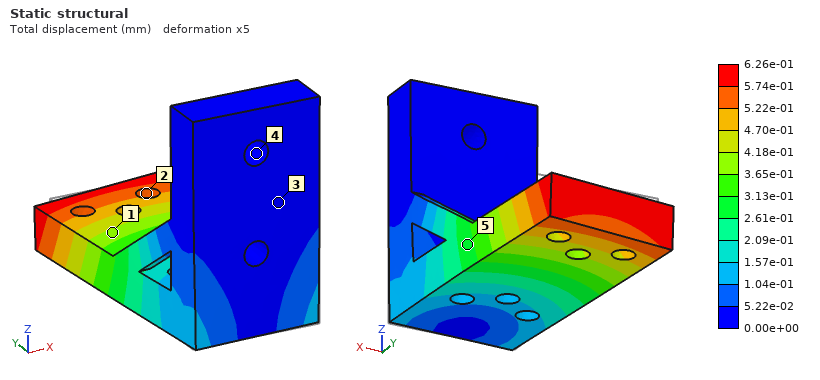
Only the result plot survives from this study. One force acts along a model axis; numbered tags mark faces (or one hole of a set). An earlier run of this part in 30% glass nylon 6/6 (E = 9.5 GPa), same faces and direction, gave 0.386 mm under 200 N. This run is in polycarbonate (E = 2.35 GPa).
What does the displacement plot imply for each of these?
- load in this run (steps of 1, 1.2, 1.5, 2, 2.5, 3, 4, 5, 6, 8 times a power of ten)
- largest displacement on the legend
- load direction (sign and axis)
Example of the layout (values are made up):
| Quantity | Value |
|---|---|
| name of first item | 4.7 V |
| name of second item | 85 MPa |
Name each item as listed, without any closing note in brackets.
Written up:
| Quantity | Value |
|---|---|
| load in this run | 80 N |
| largest displacement on the legend | 6.26e-01 mm |
| load direction | -X |
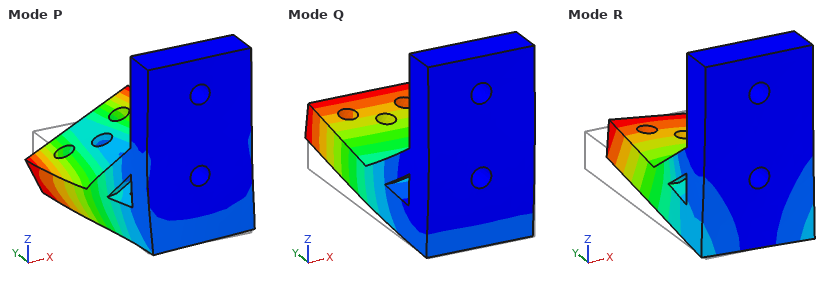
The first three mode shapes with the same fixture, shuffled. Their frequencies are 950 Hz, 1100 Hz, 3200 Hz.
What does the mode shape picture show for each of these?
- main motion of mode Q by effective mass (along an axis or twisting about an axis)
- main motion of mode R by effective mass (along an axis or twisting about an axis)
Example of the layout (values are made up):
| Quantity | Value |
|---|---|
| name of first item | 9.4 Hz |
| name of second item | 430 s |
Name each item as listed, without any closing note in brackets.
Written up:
| Quantity | Value |
|---|---|
| main motion of mode Q by effective mass | along Z |
| main motion of mode R by effective mass | along X |
